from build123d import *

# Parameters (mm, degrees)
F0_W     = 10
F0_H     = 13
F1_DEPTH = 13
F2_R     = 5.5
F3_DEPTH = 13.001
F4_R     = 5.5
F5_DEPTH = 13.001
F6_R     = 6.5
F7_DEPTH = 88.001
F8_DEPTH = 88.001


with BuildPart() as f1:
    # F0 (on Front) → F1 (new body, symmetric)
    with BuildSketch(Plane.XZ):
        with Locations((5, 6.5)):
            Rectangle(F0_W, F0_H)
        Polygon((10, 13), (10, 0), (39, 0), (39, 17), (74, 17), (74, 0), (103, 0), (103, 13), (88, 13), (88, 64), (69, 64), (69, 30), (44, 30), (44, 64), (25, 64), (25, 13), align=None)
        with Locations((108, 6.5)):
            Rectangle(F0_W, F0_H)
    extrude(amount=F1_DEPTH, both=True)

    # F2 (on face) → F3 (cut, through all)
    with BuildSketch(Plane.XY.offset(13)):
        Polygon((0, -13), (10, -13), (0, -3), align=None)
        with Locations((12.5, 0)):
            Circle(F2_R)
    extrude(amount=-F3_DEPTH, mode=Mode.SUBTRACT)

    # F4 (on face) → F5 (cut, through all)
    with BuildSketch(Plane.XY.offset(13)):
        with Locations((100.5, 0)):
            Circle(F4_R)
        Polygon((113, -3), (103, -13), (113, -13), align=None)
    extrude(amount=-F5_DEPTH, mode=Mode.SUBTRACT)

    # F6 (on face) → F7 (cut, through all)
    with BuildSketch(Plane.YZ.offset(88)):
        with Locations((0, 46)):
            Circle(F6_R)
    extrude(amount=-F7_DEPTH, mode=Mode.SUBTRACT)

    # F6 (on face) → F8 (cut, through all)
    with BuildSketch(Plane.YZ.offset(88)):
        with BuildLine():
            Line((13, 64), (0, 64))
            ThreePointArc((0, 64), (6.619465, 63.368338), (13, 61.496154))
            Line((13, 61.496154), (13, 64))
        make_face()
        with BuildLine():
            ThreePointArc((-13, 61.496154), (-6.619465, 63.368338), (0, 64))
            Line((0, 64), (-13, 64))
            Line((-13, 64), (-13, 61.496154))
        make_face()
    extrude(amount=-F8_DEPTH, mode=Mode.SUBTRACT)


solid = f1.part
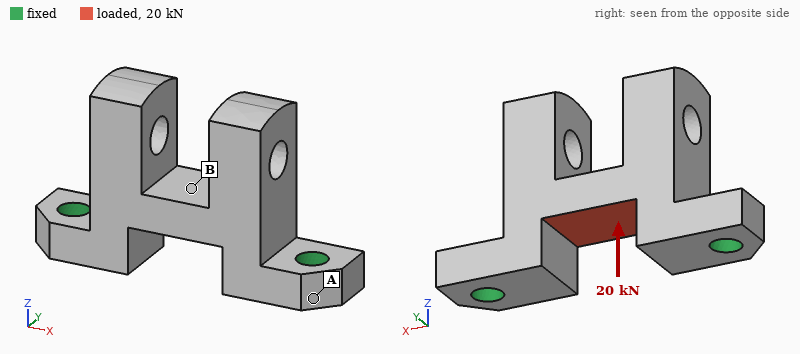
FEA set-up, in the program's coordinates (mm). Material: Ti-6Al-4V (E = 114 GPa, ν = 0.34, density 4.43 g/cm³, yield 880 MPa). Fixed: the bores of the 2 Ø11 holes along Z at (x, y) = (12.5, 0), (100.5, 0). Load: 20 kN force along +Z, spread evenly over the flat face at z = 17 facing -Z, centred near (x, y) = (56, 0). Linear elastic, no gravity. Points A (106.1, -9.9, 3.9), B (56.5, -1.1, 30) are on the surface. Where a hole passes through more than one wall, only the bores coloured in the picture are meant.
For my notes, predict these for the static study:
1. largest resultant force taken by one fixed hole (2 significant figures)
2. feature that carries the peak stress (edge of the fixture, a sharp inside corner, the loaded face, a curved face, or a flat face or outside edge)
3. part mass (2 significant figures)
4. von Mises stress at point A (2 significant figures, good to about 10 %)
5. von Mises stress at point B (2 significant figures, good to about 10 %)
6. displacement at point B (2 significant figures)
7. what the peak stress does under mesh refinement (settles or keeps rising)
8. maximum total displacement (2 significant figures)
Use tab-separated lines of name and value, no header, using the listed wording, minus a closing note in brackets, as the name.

largest resultant force taken by one fixed hole	14 kN
feature that carries the peak stress	edge of the fixture
part mass	330 g
von Mises stress at point A	25 MPa
von Mises stress at point B	110 MPa
displacement at point B	46 µm
what the peak stress does under mesh refinement	keeps rising
maximum total displacement	63 µm
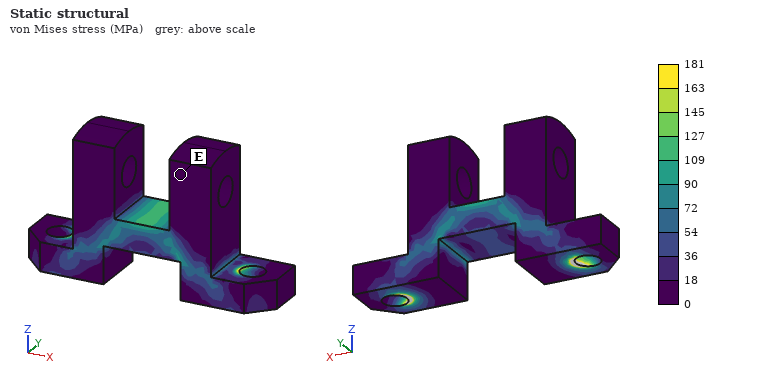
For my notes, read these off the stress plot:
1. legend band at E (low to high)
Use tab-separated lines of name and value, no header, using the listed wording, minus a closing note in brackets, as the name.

legend band at E	0 to 18 MPa
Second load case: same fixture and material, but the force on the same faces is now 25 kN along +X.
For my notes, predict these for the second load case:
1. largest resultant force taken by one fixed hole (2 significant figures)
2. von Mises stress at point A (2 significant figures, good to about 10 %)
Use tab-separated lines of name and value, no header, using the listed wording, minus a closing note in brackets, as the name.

largest resultant force taken by one fixed hole	13 kN
von Mises stress at point A	18 MPa
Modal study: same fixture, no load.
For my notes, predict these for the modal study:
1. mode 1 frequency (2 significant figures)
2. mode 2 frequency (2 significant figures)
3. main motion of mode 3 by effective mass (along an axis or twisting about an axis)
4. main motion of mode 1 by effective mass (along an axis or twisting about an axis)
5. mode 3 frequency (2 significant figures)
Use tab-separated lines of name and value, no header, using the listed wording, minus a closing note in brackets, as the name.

mode 1 frequency	2700 Hz
mode 2 frequency	4300 Hz
main motion of mode 3 by effective mass	along X
main motion of mode 1 by effective mass	along Y
mode 3 frequency	5700 Hz
